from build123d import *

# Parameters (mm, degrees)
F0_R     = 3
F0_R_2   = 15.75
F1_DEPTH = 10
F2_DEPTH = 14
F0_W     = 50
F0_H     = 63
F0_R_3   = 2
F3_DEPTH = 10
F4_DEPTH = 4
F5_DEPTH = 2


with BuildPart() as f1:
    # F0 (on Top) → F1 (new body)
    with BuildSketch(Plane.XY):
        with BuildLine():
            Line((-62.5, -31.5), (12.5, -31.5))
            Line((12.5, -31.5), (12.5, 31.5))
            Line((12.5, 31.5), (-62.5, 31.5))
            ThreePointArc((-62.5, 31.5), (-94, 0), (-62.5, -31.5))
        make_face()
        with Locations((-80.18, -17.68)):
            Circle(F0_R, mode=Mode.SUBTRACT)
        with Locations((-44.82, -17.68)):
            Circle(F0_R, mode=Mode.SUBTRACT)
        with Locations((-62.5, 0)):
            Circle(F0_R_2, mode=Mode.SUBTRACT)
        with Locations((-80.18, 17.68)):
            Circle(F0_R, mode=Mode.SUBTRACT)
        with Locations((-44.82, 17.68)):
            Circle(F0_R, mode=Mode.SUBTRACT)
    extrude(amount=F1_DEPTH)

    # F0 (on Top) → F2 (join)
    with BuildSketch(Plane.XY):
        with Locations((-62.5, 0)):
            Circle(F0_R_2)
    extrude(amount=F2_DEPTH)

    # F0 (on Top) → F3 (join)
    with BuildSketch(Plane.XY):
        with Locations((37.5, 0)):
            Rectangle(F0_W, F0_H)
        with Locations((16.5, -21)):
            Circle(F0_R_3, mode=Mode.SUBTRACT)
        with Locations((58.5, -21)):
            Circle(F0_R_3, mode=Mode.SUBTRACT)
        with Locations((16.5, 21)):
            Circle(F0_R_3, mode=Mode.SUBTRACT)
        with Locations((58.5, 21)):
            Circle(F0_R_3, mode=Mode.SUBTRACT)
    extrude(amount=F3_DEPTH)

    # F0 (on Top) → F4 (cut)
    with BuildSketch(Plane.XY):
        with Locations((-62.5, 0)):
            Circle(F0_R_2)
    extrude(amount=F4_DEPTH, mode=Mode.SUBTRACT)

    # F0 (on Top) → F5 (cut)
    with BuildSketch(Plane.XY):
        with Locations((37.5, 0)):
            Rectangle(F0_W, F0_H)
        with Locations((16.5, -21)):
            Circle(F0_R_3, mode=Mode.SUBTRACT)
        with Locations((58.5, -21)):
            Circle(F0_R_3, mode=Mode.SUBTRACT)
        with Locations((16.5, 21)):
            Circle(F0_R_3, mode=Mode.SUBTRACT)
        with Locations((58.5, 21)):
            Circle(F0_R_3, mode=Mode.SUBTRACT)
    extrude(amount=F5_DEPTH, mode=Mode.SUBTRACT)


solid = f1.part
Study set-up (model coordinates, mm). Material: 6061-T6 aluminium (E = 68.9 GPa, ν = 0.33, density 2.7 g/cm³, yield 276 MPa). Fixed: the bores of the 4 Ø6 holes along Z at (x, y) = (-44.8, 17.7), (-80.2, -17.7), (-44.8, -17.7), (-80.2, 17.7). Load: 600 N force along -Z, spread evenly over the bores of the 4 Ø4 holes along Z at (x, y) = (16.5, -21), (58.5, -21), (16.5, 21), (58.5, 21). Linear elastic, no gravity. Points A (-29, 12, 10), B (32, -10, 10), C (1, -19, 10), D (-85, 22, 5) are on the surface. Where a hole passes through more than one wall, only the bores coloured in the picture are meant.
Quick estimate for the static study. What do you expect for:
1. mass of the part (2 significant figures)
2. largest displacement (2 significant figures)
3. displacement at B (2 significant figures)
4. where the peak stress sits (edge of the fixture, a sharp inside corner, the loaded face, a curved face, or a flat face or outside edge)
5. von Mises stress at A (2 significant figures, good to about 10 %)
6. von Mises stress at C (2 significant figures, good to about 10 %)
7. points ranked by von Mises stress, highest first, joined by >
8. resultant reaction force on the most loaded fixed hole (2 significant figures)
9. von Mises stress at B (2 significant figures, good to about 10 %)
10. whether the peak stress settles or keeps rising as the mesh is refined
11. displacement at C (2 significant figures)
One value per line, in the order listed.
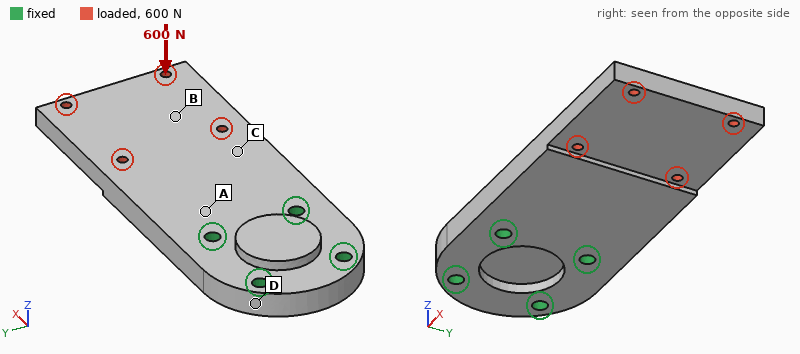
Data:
230 g
0.50 mm
0.30 mm
edge of the fixture
35 MPa
21 MPa
A > C > B > D
510 N
11 MPa
keeps rising
0.12 mm
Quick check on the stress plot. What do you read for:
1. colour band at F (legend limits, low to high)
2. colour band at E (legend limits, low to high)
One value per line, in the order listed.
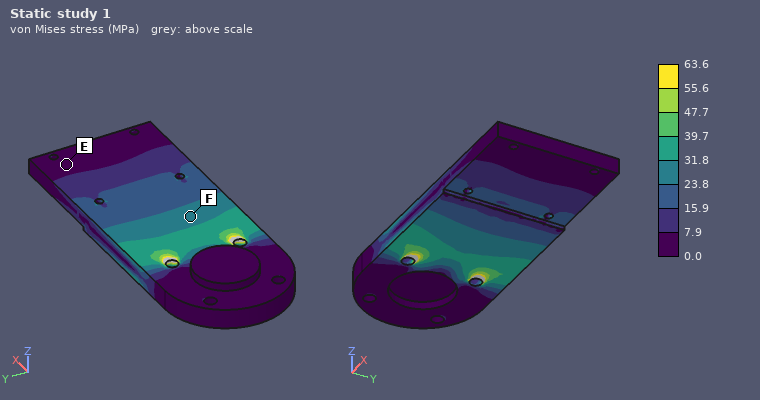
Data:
23.8 to 31.8 MPa
0.0 to 7.9 MPa
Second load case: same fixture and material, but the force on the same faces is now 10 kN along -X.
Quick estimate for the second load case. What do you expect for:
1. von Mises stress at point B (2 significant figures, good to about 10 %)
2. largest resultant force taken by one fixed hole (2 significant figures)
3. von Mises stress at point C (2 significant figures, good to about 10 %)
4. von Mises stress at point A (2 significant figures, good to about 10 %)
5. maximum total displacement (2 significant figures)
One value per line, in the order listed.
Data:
12 MPa
4.3 kN
27 MPa
26 MPa
0.12 mm
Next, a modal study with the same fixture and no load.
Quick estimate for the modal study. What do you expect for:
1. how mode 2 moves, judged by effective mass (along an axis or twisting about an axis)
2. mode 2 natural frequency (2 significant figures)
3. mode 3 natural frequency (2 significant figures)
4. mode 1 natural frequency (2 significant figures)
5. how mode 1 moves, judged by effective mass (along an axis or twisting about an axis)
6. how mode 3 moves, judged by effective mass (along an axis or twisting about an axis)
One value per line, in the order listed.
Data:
twisting about X
2500 Hz
3700 Hz
760 Hz
along Z
along Y
